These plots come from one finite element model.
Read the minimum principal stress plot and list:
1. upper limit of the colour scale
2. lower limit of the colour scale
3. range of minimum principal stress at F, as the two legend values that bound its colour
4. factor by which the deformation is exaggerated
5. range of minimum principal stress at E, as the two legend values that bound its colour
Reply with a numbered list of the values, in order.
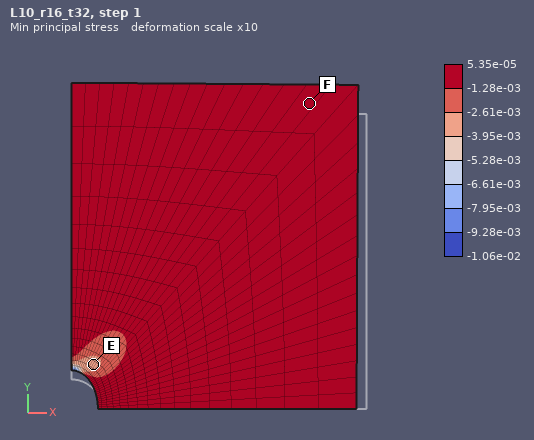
1. 5.35e-05
2. -1.06e-02
3. -1.28e-03 to 5.35e-05
4. 10
5. -3.95e-03 to -2.61e-03
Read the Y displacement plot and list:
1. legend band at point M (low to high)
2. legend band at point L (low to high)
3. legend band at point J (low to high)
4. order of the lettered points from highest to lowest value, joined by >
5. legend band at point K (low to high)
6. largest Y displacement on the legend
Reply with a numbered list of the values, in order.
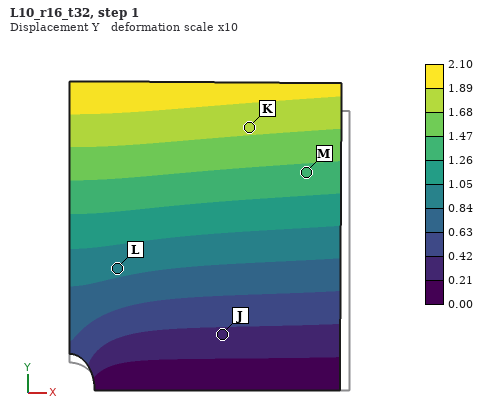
1. 1.26 to 1.47
2. 0.84 to 1.05
3. 0.21 to 0.42
4. K > M > L > J
5. 1.68 to 1.89
6. 2.10
